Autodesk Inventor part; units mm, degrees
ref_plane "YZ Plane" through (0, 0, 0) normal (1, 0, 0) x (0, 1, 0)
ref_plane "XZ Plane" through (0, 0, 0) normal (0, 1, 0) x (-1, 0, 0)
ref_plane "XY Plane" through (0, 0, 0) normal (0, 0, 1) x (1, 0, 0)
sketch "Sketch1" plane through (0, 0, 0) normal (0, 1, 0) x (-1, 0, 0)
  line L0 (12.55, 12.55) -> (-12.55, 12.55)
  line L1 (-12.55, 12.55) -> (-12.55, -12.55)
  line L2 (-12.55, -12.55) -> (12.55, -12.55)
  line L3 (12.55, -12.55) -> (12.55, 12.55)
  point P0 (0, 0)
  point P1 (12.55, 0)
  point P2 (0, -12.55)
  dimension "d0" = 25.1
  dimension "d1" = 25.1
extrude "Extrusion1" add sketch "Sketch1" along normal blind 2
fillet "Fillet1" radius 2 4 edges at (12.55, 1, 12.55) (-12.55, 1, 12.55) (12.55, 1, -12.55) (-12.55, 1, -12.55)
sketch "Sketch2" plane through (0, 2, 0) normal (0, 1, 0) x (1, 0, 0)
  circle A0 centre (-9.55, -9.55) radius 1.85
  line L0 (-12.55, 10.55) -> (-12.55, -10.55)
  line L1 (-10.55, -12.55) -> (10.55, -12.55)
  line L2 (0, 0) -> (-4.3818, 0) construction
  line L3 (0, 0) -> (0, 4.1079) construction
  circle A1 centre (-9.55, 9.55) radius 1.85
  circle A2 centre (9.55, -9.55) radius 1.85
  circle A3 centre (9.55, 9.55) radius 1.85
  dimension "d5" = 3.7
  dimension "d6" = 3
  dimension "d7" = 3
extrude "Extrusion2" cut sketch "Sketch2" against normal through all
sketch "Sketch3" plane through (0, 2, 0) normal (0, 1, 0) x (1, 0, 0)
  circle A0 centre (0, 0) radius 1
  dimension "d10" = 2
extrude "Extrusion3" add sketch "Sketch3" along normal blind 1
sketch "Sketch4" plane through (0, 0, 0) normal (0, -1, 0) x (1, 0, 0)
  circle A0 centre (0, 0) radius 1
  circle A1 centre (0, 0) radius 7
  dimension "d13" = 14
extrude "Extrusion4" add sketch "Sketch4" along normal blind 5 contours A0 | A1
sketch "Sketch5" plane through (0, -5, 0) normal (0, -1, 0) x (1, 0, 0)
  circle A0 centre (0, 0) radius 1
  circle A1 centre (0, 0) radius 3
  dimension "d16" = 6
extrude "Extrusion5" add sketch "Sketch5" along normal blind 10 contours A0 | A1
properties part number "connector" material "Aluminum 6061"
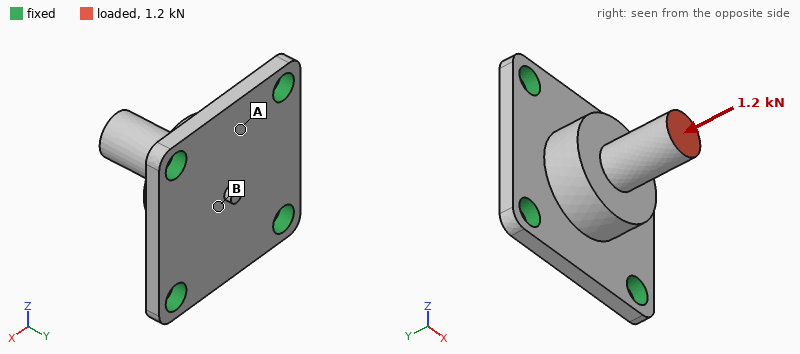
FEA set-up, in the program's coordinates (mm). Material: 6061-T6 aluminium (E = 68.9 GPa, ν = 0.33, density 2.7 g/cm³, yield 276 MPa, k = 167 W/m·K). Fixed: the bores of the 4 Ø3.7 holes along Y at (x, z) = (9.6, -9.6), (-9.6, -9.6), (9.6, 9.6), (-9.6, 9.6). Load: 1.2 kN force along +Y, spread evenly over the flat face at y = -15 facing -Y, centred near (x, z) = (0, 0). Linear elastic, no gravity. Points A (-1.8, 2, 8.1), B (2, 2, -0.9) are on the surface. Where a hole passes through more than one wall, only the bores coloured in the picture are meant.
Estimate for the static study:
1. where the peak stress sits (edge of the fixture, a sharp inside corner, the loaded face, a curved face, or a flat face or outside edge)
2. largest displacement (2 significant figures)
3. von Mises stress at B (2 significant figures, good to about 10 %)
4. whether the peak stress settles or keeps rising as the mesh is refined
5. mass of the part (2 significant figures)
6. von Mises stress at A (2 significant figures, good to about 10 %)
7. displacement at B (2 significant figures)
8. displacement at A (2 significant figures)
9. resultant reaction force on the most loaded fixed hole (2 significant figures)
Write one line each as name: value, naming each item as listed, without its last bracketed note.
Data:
where the peak stress sits: edge of the fixture
largest displacement: 28 µm
von Mises stress at B: 22 MPa
whether the peak stress settles or keeps rising as the mesh is refined: keeps rising
mass of the part: 6.0 g
von Mises stress at A: 44 MPa
displacement at B: 21 µm
displacement at A: 16 µm
resultant reaction force on the most loaded fixed hole: 320 N
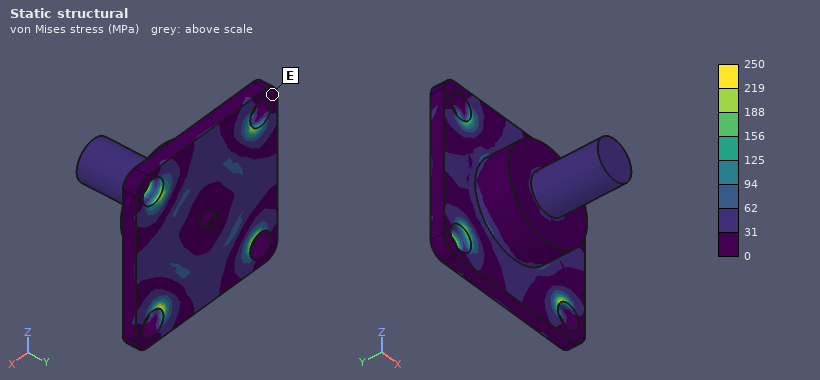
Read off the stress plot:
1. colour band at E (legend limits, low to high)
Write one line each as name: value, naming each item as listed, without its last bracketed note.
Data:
colour band at E: 0 to 31 MPa
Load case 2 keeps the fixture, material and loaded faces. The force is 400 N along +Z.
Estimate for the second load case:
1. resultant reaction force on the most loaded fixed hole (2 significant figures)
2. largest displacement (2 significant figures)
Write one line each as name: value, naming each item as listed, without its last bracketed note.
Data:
resultant reaction force on the most loaded fixed hole: 240 N
largest displacement: 86 µm
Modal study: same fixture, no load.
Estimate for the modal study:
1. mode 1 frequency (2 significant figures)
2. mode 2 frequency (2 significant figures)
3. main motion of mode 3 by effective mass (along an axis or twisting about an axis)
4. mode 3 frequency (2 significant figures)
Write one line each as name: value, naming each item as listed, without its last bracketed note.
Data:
mode 1 frequency: 18 kHz
mode 2 frequency: 18 kHz
main motion of mode 3 by effective mass: along Y
mode 3 frequency: 19 kHz
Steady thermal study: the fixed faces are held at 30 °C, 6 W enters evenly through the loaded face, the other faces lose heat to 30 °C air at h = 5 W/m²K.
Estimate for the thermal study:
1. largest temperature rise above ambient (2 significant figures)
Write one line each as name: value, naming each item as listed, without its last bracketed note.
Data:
largest temperature rise above ambient: 18 K
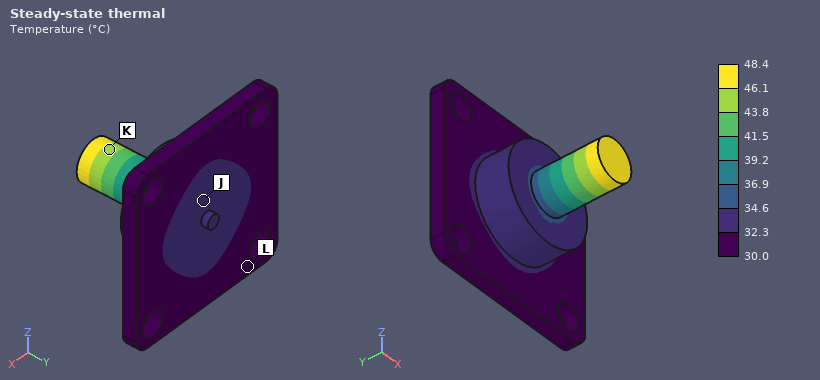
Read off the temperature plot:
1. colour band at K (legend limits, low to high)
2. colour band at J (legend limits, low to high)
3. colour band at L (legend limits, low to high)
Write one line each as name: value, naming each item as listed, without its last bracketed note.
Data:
colour band at K: 43.8 to 46.1 °C
colour band at J: 32.3 to 34.6 °C
colour band at L: 30.0 to 32.3 °C
